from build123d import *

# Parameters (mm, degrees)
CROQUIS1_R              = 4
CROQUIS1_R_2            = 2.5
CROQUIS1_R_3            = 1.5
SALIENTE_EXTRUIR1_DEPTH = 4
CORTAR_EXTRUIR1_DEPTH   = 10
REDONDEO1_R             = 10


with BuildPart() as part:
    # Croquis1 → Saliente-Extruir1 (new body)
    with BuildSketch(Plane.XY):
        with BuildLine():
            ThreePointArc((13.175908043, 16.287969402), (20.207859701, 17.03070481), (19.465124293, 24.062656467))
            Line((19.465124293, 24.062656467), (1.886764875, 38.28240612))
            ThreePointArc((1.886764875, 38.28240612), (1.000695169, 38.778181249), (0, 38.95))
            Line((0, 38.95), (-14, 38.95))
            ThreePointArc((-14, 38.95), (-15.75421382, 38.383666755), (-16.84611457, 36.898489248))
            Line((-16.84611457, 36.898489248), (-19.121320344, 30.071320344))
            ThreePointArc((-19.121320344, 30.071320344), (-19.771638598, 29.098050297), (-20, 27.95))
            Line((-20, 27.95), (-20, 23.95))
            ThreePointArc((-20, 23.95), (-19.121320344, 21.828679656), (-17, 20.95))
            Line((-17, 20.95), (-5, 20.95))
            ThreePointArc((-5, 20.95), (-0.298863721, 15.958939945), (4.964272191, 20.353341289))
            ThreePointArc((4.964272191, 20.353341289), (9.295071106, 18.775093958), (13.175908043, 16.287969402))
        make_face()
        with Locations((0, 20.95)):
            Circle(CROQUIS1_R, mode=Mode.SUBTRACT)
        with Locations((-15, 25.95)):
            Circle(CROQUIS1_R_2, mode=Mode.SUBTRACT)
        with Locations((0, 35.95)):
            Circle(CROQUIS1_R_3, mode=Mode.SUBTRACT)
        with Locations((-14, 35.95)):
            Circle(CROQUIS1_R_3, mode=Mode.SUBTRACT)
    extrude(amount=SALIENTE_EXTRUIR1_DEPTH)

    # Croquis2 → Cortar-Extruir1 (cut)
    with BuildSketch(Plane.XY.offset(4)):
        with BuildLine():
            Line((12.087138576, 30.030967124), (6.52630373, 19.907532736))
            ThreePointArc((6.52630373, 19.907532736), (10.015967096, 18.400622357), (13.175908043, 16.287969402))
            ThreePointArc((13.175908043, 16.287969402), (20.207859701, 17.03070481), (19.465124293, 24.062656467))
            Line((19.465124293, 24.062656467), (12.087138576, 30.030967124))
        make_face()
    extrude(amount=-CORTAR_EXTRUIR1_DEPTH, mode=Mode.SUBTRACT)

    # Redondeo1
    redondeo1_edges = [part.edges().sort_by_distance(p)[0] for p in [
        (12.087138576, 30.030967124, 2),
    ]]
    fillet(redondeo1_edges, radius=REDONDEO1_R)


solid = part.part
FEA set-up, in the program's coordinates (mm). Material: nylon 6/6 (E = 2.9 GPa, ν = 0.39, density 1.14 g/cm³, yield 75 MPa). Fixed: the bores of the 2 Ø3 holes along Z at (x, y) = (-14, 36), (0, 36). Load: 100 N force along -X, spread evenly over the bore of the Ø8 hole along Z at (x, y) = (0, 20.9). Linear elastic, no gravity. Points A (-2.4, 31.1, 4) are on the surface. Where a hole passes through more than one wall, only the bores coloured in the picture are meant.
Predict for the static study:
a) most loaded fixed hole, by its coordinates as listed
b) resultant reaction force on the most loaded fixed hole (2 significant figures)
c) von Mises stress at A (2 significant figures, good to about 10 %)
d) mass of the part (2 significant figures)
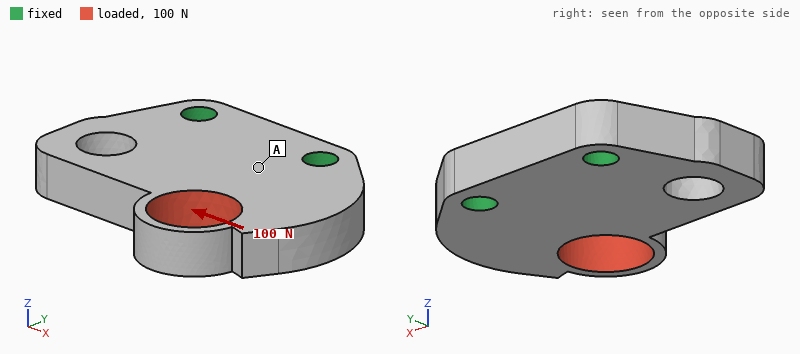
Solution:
(-14, 36)
110 N
3.9 MPa
1.9 g
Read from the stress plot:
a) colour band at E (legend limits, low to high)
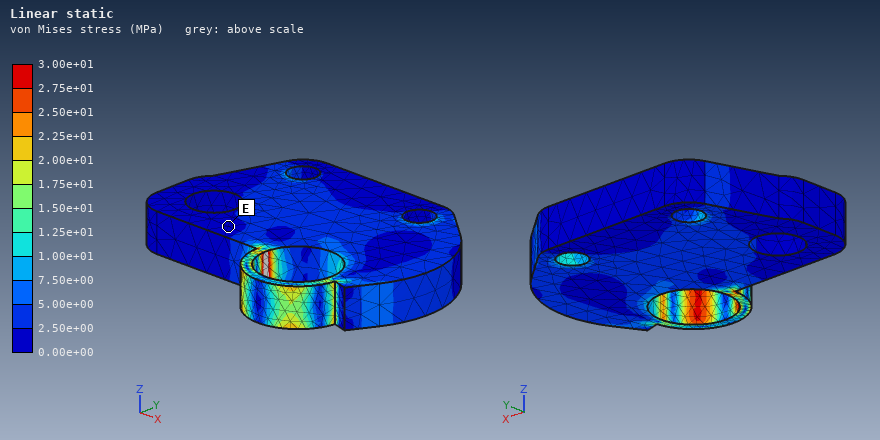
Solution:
0.00e+00 to 2.50e+00 MPa
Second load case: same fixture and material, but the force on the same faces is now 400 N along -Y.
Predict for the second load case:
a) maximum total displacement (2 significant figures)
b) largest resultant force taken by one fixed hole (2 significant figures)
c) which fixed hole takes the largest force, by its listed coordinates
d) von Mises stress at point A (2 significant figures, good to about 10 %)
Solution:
0.18 mm
370 N
(0, 36)
8.6 MPa
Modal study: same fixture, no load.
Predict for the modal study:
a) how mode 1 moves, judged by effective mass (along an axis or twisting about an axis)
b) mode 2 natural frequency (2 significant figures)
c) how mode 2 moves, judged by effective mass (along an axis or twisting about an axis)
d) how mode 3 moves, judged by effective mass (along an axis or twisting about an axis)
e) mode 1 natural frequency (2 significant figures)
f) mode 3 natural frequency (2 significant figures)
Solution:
along Z
5600 Hz
twisting about Y
along X
3900 Hz
9100 Hz
